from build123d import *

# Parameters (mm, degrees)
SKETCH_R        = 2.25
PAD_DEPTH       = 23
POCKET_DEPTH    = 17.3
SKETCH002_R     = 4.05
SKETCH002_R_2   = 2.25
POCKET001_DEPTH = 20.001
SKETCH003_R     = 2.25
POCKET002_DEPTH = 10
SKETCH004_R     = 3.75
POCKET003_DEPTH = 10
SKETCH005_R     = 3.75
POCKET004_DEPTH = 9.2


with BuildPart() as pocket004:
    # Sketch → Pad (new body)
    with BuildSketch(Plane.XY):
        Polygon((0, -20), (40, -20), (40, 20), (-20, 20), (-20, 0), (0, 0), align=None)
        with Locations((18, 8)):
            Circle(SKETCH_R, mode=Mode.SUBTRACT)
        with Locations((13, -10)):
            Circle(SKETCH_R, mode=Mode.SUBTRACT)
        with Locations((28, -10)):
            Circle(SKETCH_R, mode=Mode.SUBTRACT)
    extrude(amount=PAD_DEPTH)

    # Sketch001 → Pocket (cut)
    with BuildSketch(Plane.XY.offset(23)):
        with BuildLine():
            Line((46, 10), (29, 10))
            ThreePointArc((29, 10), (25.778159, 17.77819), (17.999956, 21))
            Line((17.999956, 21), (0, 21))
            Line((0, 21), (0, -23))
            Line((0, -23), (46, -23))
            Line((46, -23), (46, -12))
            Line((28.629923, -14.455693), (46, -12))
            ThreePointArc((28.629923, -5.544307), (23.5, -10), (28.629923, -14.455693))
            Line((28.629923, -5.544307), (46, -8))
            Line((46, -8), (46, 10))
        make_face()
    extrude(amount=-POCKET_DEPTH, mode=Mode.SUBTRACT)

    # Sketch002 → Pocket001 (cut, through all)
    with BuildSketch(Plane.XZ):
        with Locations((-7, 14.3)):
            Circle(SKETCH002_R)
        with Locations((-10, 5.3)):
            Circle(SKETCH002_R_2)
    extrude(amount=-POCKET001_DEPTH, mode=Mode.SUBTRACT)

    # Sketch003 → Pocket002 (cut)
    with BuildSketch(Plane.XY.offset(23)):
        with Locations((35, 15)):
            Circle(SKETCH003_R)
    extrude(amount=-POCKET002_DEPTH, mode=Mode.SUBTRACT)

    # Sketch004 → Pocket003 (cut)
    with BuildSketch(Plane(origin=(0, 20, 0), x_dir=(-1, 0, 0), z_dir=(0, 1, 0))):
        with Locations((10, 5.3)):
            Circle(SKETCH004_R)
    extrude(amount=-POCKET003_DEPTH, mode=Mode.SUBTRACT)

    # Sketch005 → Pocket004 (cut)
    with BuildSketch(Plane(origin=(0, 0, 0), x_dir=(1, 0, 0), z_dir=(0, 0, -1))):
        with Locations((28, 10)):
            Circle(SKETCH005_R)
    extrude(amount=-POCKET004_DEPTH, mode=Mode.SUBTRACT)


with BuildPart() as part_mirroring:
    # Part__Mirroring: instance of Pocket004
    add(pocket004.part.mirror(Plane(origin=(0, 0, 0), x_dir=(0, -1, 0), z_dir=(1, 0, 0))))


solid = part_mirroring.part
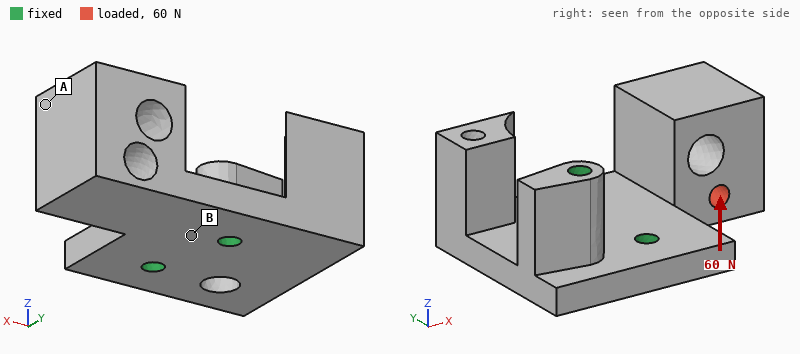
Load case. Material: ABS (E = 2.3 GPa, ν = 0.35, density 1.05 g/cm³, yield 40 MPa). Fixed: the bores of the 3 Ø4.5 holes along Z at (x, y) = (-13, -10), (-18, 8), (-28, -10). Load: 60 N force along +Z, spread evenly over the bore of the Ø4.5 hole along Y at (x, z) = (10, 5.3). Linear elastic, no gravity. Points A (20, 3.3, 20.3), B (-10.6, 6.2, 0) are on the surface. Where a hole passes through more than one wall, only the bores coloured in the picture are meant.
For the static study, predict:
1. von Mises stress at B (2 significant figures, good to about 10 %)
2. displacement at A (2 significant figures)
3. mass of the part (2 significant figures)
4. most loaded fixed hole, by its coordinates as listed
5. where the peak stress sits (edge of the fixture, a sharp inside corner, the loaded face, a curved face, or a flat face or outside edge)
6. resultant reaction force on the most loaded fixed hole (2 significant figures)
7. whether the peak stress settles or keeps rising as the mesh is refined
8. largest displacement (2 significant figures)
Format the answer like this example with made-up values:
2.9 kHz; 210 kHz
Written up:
6.5 MPa; 0.66 mm; 21 g; (-13, -10); edge of the fixture; 42 N; keeps rising; 0.71 mm
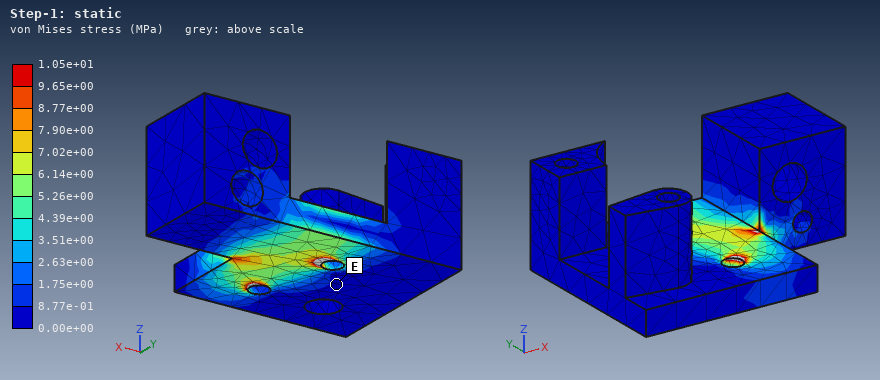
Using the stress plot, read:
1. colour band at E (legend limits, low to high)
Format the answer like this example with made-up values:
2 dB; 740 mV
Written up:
0.00e+00 to 8.77e-01 MPa
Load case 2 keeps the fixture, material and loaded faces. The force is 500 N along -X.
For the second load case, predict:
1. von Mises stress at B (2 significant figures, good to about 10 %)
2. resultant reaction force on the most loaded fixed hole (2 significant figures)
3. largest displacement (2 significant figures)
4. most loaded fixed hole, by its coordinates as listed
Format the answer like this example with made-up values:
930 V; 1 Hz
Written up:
4.3 MPa; 400 N; 0.85 mm; (-18, 8)
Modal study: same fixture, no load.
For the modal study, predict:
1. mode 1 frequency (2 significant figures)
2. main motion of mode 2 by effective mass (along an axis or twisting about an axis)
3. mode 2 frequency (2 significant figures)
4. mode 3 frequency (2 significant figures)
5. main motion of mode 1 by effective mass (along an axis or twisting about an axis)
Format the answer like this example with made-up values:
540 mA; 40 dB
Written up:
560 Hz; along Y; 1300 Hz; 1600 Hz; along Z
